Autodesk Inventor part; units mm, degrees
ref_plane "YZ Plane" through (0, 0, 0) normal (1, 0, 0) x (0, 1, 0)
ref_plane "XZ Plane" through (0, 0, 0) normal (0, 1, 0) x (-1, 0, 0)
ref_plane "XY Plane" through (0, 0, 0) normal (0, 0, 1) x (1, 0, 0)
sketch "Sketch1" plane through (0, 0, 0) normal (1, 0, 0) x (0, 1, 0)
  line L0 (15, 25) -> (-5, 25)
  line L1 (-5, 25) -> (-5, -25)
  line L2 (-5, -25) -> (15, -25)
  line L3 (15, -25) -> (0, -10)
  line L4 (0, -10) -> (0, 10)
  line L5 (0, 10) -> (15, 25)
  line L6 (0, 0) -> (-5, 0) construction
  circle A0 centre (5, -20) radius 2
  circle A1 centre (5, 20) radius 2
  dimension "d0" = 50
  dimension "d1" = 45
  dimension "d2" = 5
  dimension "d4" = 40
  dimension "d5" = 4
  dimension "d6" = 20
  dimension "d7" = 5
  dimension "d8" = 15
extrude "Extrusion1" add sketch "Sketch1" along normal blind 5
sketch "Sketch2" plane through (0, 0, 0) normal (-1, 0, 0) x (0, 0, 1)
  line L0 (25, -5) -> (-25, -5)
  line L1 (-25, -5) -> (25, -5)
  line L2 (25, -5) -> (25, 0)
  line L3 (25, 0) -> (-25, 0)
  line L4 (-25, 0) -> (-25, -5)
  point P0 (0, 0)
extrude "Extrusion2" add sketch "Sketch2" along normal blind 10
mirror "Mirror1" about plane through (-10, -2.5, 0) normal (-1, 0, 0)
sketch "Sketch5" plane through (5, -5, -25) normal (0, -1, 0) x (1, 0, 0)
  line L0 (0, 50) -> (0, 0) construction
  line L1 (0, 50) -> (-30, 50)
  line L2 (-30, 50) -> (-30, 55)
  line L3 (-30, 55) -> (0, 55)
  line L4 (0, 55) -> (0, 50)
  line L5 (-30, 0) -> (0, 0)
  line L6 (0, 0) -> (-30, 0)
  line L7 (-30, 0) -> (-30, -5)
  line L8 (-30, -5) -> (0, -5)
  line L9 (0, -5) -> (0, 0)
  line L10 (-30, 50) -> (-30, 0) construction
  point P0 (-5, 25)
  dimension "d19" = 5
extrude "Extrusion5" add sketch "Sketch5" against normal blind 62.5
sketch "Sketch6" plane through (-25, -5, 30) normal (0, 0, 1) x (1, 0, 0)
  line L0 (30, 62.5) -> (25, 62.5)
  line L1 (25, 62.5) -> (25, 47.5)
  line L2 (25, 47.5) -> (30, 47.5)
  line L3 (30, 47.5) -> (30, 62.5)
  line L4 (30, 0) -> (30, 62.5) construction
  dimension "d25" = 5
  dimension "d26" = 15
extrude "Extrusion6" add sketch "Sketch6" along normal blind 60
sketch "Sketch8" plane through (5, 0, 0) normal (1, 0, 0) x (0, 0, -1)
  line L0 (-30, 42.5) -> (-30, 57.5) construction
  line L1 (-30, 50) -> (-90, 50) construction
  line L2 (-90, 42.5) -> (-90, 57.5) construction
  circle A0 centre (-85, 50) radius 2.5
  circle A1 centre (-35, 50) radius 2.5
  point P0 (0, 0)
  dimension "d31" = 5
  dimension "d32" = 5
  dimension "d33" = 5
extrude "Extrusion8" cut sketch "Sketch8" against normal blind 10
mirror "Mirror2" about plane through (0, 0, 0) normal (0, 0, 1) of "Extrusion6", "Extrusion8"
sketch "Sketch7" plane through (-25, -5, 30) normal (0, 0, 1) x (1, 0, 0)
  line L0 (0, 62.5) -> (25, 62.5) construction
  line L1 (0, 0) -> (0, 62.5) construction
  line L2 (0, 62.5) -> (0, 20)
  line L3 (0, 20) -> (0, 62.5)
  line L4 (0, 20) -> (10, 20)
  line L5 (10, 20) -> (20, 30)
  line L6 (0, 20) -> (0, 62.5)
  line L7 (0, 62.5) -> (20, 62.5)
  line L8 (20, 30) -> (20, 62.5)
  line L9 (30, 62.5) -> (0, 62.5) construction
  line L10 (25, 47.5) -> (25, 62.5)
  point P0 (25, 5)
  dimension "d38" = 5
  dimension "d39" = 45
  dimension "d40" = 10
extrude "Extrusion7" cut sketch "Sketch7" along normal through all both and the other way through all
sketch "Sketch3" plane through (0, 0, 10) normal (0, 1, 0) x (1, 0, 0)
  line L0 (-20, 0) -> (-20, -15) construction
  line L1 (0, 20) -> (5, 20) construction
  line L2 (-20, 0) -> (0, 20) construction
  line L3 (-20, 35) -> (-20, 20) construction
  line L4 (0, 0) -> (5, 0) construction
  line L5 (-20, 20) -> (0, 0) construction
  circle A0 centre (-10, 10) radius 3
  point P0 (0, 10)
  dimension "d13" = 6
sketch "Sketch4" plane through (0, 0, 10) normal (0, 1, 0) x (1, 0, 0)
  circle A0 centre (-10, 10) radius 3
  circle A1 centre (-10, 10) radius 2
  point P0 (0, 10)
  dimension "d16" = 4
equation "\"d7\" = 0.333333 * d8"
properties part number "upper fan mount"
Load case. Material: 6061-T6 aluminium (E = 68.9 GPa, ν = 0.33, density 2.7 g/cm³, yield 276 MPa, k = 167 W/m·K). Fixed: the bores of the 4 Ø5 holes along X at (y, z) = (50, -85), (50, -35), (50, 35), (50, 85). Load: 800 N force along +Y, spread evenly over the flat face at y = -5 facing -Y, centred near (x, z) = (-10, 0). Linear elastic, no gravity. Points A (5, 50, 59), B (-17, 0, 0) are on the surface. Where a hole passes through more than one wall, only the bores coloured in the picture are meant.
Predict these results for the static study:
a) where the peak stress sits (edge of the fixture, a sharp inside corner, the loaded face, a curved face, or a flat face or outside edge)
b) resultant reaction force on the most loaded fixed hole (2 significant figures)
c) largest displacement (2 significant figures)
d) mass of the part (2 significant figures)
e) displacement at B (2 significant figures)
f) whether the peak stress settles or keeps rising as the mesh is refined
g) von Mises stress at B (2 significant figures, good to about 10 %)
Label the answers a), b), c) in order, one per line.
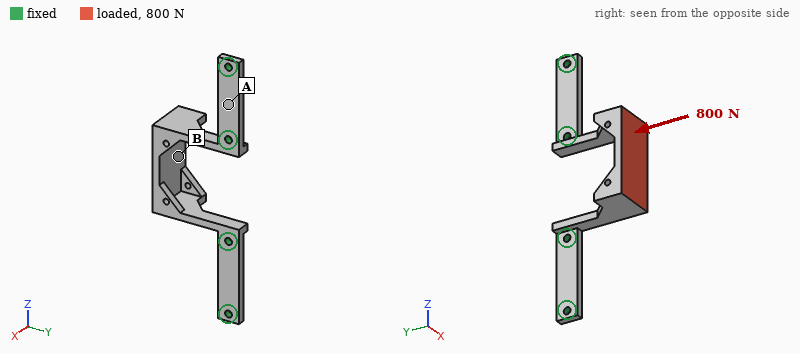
a) edge of the fixture
b) 420 N
c) 0.32 mm
d) 78 g
e) 0.26 mm
f) keeps rising
g) 19 MPa
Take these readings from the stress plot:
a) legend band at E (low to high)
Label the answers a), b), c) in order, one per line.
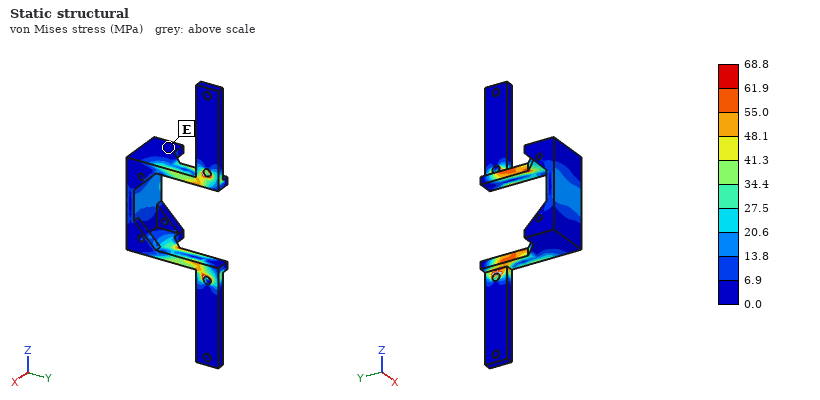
a) 0.0 to 6.9 MPa
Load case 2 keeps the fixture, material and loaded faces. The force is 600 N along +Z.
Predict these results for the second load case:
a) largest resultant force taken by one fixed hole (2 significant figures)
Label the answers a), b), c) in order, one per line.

a) 450 N
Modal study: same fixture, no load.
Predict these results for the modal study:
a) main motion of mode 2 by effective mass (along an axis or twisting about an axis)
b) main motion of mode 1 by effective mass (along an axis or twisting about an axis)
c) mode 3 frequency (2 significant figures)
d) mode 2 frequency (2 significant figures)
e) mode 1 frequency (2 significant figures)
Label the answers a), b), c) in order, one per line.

a) along Z
b) along X
c) 1900 Hz
d) 1300 Hz
e) 730 Hz
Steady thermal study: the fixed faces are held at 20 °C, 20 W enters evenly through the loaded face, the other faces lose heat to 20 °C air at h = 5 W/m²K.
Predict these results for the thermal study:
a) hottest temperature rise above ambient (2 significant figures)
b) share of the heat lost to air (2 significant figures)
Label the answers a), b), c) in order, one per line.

a) 48 K
b) 7.4 %
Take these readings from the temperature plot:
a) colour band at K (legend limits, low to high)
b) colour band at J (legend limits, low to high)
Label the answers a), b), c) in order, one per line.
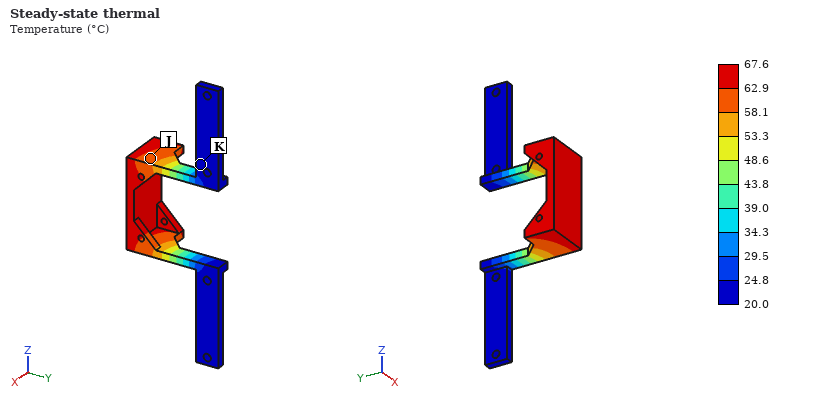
a) 20.0 to 24.8 °C
b) 58.1 to 62.9 °C
